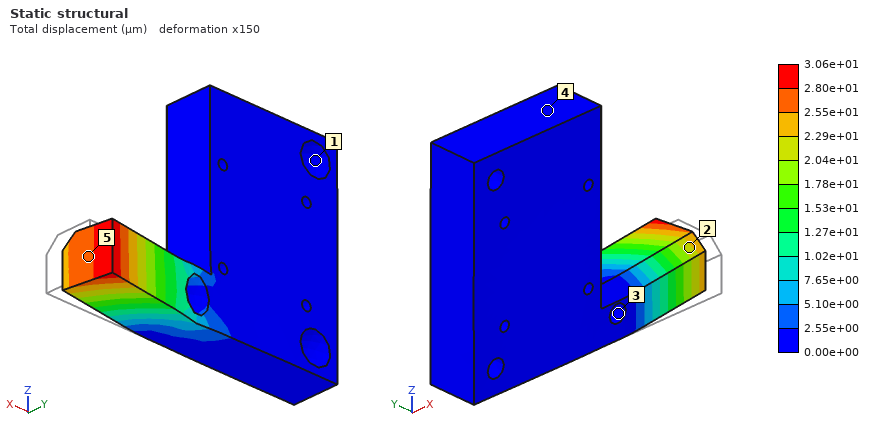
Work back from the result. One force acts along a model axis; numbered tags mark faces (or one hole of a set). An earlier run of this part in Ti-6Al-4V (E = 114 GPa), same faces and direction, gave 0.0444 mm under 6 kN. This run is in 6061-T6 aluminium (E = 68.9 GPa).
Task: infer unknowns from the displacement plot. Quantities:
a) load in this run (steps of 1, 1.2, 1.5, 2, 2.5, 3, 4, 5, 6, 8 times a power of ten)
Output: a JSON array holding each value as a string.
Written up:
["2.5 kN"]
